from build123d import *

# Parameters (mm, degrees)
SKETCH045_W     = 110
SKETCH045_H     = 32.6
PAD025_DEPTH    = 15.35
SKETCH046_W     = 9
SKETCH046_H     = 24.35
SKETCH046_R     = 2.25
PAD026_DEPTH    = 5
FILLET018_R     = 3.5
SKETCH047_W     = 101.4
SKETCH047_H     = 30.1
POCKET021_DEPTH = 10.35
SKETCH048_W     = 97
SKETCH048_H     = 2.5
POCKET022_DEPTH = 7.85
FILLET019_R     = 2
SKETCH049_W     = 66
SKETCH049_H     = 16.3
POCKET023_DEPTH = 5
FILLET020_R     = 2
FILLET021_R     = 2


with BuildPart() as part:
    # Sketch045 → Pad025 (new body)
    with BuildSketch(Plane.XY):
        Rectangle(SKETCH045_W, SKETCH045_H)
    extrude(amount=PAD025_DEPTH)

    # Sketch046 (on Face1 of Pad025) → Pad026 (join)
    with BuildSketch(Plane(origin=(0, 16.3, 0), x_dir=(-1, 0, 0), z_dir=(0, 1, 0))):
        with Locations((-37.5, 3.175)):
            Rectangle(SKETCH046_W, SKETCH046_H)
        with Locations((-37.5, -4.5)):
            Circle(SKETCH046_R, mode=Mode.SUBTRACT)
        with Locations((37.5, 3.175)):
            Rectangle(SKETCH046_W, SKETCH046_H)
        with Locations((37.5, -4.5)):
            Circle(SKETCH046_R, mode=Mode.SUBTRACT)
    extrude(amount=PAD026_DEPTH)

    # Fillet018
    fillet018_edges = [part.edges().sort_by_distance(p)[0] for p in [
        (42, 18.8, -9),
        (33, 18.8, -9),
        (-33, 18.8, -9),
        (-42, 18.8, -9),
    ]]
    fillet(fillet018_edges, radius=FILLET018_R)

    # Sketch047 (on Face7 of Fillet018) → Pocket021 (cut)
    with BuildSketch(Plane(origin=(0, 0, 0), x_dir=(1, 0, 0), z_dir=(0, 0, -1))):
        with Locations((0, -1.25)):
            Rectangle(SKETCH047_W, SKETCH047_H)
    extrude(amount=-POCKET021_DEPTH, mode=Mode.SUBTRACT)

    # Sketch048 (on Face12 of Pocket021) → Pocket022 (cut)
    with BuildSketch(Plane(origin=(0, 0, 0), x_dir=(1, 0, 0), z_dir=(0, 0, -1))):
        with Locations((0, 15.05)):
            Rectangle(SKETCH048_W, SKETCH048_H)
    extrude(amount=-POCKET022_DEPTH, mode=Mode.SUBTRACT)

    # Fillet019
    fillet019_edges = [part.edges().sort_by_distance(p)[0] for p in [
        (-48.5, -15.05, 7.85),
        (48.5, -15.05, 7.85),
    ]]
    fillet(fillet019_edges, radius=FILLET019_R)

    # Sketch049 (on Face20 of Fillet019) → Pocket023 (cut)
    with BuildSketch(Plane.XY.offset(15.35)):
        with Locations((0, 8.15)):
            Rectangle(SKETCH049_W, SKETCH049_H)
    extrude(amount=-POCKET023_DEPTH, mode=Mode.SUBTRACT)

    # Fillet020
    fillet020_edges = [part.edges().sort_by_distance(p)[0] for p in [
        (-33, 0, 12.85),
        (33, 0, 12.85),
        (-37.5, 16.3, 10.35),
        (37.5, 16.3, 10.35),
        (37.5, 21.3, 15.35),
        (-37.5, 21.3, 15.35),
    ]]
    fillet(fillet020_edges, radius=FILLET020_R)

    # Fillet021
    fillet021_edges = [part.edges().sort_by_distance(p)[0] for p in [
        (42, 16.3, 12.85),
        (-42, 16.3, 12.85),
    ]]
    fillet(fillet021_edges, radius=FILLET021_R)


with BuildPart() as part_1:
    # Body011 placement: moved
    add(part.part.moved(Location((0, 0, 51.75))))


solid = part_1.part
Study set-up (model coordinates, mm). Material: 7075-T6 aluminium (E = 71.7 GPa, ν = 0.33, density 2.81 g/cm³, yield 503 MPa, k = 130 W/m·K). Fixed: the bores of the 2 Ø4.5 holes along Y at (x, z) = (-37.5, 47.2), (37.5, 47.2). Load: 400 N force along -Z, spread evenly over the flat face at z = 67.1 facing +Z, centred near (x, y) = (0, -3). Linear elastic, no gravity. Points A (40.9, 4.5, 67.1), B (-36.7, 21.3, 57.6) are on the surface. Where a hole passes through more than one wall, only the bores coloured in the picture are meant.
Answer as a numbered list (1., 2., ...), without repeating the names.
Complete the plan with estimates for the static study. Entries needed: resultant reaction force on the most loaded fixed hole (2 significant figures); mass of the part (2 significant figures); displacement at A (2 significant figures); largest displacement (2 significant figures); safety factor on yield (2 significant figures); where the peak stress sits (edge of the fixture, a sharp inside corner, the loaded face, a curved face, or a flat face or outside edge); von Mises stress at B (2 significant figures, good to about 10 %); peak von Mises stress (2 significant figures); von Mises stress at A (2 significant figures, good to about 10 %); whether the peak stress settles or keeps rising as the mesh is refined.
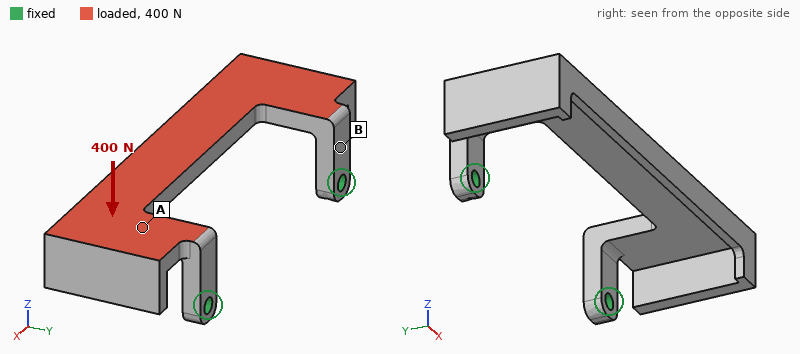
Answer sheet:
1. 200 N
2. 51 g
3. 0.20 mm
4. 0.48 mm
5. 2.8
6. a flat face or outside edge
7. 110 MPa
8. 180 MPa
9. 17 MPa
10. settles
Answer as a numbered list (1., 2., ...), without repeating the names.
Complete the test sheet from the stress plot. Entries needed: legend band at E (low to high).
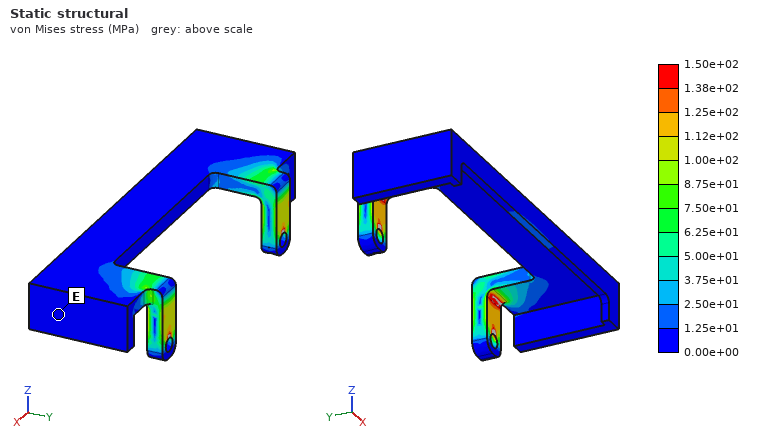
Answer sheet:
1. 0.00e+00 to 1.25e+01 MPa
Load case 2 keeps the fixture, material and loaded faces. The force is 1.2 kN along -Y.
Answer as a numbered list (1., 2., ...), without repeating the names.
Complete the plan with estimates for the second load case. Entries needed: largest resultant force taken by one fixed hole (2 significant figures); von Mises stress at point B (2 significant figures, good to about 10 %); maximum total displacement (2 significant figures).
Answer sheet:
1. 600 N
2. 150 MPa
3. 0.61 mm
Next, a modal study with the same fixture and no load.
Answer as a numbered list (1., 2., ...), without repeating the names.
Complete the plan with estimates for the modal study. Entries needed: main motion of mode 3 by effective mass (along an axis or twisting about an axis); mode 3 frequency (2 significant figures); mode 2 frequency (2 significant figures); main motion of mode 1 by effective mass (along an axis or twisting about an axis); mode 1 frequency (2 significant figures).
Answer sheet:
1. along X
2. 2200 Hz
3. 1400 Hz
4. along Z
5. 790 Hz
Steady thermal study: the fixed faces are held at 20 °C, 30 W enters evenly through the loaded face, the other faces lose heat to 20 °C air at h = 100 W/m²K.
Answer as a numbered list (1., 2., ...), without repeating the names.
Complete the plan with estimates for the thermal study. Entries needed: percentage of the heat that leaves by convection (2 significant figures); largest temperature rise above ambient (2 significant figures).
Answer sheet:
1. 58 %
2. 33 K
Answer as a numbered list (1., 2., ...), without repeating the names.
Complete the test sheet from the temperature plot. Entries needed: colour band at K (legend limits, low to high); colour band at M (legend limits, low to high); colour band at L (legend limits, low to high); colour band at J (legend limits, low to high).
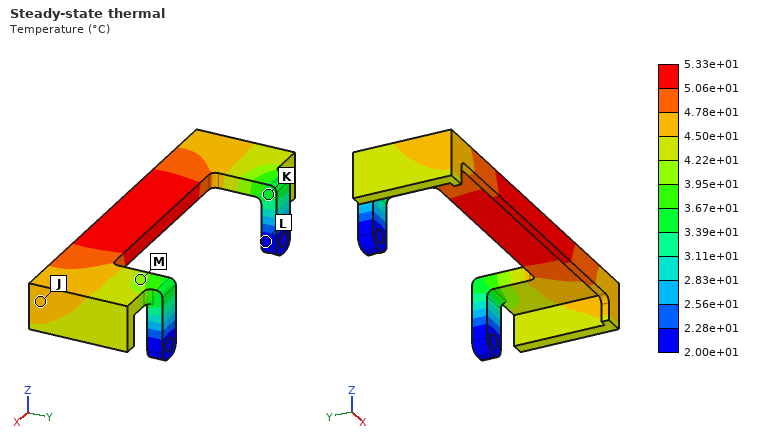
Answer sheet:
1. 3.39e+01 to 3.67e+01 °C
2. 3.95e+01 to 4.22e+01 °C
3. 2.00e+01 to 2.28e+01 °C
4. 4.50e+01 to 4.78e+01 °C
